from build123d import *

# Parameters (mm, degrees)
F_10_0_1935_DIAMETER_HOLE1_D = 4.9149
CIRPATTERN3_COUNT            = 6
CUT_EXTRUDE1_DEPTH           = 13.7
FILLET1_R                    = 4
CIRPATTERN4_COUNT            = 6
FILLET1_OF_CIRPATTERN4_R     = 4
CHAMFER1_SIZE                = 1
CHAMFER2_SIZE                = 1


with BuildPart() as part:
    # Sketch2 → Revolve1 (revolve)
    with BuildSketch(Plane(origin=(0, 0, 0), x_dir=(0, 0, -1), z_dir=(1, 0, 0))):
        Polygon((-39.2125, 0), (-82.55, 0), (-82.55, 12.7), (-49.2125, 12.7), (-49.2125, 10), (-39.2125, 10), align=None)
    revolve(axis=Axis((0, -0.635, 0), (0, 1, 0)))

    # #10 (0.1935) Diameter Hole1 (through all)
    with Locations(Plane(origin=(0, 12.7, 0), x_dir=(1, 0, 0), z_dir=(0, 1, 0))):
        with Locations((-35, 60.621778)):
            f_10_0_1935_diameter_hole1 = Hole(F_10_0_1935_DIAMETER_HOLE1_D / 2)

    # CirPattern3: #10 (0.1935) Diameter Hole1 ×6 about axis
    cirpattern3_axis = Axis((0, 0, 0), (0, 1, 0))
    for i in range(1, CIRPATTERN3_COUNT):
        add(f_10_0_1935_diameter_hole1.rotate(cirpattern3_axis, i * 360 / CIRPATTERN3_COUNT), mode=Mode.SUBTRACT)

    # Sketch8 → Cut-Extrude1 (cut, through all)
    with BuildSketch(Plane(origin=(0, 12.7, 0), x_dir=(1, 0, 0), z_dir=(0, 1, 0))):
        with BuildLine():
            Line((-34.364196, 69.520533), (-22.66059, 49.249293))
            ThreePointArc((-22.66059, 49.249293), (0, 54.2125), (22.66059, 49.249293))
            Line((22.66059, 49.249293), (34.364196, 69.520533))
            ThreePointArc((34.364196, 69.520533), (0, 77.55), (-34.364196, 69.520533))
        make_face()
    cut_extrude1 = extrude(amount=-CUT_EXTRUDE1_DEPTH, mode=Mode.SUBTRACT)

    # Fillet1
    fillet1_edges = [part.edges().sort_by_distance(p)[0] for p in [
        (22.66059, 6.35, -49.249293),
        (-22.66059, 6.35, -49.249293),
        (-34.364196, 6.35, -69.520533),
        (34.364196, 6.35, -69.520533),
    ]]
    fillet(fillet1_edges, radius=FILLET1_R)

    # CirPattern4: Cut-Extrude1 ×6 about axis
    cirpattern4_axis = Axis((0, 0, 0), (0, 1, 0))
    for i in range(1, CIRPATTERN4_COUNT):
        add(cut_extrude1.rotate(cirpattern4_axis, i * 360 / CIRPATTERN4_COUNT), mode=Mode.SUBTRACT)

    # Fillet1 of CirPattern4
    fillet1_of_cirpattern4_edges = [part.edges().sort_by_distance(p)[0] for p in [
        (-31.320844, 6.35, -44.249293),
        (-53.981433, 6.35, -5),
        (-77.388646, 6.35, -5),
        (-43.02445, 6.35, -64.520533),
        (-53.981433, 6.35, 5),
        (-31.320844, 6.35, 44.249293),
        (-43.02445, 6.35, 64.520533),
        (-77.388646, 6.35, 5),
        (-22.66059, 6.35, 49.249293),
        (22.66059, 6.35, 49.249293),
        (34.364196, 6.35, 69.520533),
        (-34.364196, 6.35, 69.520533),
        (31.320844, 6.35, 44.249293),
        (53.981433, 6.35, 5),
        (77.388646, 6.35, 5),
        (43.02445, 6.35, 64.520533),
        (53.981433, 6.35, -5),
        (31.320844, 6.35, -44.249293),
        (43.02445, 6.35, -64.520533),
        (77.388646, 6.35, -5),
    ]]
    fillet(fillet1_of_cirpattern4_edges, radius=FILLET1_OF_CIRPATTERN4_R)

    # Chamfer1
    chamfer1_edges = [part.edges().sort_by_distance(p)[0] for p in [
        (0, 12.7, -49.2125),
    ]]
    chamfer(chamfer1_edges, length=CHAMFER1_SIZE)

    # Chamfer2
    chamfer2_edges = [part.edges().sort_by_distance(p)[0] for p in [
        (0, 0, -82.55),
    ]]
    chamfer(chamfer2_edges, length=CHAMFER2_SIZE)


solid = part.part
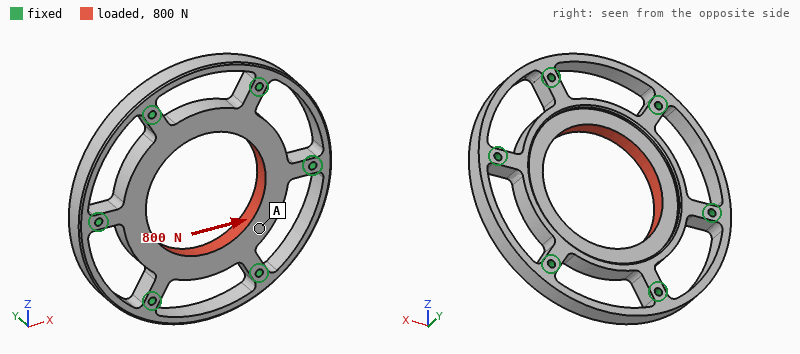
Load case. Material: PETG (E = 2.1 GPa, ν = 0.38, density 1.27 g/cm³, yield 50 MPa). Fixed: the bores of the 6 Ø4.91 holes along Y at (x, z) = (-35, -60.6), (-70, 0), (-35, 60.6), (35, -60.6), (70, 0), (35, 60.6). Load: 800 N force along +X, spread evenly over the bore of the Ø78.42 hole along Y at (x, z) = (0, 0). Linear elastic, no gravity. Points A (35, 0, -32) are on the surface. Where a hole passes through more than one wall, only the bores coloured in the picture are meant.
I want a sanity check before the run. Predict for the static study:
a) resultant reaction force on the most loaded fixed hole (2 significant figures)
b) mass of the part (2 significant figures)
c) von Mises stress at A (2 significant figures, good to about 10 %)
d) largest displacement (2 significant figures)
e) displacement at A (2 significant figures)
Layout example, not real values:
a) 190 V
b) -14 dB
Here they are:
a) 210 N
b) 120 g
c) 0.31 MPa
d) 38 µm
e) 35 µm
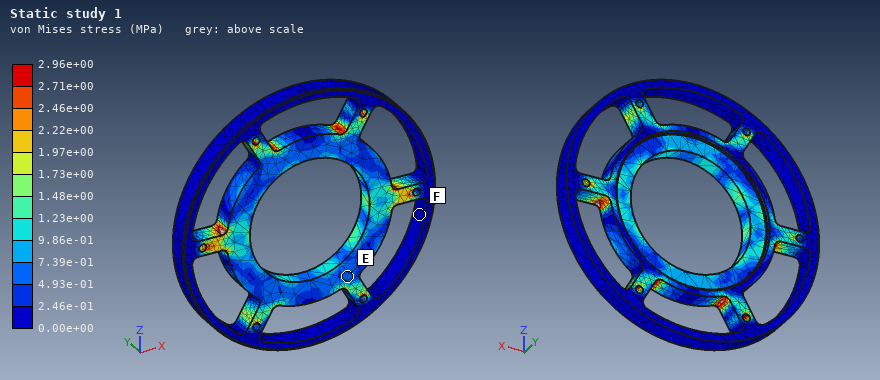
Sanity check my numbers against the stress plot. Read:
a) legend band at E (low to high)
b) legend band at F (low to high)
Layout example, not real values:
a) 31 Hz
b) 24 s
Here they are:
a) 4.93e-01 to 7.39e-01 MPa
b) 0.00e+00 to 2.46e-01 MPa
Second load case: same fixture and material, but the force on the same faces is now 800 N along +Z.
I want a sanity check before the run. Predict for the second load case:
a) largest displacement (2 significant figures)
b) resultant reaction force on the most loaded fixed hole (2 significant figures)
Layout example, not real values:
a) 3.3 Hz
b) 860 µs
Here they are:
a) 41 µm
b) 190 N
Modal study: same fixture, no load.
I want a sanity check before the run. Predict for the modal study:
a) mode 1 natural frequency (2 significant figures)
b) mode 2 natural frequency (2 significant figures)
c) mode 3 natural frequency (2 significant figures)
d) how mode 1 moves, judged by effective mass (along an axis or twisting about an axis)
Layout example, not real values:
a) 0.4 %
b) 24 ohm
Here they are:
a) 1500 Hz
b) 1600 Hz
c) 1700 Hz
d) along Y
